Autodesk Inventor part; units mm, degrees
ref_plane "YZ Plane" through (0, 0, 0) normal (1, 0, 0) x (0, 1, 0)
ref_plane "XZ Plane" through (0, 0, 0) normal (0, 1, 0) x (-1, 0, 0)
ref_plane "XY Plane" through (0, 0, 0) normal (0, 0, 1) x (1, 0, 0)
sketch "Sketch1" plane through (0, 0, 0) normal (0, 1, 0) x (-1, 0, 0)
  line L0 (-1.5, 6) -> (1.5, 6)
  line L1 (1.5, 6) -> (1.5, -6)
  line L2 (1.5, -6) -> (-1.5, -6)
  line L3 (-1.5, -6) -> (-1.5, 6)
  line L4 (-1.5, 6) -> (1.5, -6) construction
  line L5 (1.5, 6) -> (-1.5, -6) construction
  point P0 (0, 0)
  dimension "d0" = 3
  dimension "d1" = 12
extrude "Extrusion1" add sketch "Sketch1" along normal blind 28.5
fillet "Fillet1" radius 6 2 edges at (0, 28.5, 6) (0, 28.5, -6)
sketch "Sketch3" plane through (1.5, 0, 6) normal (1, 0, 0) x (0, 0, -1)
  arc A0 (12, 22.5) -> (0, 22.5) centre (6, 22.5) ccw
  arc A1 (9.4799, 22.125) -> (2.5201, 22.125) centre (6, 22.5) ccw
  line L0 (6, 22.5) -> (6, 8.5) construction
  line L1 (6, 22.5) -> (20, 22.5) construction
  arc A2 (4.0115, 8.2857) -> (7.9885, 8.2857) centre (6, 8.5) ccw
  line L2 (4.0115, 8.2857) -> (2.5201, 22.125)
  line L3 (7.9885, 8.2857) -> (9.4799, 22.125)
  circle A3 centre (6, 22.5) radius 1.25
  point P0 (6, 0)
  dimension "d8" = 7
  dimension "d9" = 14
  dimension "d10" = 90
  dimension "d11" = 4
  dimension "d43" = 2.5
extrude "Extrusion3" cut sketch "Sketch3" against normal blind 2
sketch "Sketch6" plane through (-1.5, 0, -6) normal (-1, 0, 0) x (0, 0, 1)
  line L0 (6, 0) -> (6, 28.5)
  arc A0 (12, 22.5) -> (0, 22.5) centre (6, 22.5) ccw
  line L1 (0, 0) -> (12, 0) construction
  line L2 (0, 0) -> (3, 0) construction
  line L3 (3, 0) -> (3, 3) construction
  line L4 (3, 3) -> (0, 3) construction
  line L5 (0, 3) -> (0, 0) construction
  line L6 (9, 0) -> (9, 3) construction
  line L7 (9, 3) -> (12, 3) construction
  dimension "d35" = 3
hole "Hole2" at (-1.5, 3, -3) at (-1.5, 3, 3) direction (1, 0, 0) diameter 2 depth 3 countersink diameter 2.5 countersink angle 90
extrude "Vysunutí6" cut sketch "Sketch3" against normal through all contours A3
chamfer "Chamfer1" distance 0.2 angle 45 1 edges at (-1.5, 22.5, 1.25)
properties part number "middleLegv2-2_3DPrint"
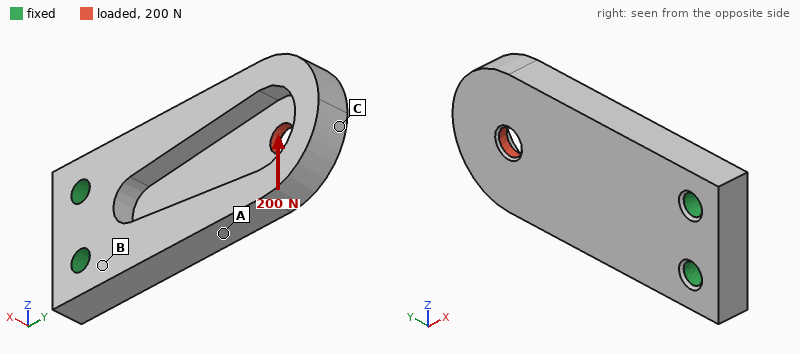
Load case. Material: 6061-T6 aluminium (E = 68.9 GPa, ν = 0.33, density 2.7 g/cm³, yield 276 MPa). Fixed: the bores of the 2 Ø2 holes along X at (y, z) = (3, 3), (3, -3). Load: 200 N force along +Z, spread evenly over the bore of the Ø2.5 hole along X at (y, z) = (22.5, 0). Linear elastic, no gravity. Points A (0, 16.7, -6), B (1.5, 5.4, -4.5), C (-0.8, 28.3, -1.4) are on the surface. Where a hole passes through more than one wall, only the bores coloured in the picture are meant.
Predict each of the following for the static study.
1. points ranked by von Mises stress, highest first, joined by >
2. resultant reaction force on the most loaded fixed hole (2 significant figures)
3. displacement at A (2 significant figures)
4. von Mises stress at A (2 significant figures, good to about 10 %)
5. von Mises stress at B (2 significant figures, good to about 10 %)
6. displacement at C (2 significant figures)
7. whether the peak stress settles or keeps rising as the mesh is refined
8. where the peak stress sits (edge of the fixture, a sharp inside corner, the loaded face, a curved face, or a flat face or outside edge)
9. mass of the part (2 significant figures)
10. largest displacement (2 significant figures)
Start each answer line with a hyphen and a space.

- B > A > C
- 520 N
- 23 µm
- 20 MPa
- 34 MPa
- 42 µm
- keeps rising
- edge of the fixture
- 2.0 g
- 46 µm
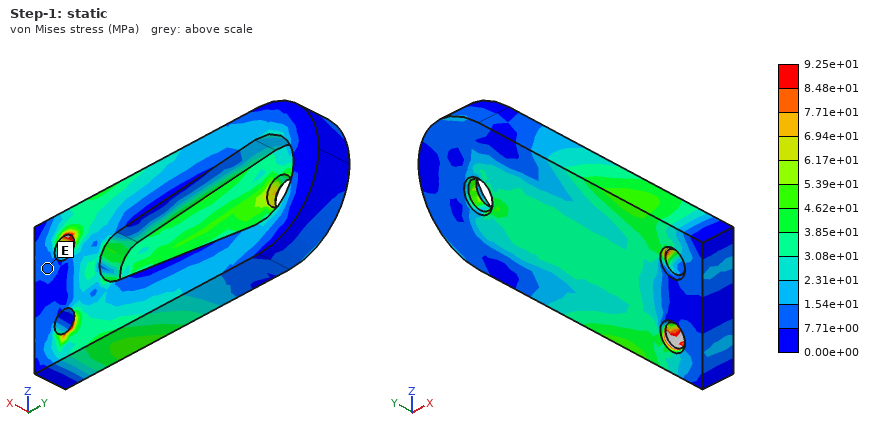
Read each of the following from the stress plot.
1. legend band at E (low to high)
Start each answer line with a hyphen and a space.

- 7.71e+00 to 1.54e+01 MPa
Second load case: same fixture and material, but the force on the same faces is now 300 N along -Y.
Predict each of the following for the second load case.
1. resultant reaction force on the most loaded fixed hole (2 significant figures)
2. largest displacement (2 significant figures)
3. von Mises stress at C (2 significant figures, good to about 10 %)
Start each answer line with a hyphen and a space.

- 150 N
- 44 µm
- 11 MPa
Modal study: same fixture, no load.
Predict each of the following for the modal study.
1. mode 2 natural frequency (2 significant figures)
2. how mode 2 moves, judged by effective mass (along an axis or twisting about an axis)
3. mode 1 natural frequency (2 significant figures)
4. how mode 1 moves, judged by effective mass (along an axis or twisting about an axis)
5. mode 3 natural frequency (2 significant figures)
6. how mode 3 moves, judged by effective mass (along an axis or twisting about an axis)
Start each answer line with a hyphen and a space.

- 11 kHz
- along Z
- 4500 Hz
- along X
- 15 kHz
- along Z
